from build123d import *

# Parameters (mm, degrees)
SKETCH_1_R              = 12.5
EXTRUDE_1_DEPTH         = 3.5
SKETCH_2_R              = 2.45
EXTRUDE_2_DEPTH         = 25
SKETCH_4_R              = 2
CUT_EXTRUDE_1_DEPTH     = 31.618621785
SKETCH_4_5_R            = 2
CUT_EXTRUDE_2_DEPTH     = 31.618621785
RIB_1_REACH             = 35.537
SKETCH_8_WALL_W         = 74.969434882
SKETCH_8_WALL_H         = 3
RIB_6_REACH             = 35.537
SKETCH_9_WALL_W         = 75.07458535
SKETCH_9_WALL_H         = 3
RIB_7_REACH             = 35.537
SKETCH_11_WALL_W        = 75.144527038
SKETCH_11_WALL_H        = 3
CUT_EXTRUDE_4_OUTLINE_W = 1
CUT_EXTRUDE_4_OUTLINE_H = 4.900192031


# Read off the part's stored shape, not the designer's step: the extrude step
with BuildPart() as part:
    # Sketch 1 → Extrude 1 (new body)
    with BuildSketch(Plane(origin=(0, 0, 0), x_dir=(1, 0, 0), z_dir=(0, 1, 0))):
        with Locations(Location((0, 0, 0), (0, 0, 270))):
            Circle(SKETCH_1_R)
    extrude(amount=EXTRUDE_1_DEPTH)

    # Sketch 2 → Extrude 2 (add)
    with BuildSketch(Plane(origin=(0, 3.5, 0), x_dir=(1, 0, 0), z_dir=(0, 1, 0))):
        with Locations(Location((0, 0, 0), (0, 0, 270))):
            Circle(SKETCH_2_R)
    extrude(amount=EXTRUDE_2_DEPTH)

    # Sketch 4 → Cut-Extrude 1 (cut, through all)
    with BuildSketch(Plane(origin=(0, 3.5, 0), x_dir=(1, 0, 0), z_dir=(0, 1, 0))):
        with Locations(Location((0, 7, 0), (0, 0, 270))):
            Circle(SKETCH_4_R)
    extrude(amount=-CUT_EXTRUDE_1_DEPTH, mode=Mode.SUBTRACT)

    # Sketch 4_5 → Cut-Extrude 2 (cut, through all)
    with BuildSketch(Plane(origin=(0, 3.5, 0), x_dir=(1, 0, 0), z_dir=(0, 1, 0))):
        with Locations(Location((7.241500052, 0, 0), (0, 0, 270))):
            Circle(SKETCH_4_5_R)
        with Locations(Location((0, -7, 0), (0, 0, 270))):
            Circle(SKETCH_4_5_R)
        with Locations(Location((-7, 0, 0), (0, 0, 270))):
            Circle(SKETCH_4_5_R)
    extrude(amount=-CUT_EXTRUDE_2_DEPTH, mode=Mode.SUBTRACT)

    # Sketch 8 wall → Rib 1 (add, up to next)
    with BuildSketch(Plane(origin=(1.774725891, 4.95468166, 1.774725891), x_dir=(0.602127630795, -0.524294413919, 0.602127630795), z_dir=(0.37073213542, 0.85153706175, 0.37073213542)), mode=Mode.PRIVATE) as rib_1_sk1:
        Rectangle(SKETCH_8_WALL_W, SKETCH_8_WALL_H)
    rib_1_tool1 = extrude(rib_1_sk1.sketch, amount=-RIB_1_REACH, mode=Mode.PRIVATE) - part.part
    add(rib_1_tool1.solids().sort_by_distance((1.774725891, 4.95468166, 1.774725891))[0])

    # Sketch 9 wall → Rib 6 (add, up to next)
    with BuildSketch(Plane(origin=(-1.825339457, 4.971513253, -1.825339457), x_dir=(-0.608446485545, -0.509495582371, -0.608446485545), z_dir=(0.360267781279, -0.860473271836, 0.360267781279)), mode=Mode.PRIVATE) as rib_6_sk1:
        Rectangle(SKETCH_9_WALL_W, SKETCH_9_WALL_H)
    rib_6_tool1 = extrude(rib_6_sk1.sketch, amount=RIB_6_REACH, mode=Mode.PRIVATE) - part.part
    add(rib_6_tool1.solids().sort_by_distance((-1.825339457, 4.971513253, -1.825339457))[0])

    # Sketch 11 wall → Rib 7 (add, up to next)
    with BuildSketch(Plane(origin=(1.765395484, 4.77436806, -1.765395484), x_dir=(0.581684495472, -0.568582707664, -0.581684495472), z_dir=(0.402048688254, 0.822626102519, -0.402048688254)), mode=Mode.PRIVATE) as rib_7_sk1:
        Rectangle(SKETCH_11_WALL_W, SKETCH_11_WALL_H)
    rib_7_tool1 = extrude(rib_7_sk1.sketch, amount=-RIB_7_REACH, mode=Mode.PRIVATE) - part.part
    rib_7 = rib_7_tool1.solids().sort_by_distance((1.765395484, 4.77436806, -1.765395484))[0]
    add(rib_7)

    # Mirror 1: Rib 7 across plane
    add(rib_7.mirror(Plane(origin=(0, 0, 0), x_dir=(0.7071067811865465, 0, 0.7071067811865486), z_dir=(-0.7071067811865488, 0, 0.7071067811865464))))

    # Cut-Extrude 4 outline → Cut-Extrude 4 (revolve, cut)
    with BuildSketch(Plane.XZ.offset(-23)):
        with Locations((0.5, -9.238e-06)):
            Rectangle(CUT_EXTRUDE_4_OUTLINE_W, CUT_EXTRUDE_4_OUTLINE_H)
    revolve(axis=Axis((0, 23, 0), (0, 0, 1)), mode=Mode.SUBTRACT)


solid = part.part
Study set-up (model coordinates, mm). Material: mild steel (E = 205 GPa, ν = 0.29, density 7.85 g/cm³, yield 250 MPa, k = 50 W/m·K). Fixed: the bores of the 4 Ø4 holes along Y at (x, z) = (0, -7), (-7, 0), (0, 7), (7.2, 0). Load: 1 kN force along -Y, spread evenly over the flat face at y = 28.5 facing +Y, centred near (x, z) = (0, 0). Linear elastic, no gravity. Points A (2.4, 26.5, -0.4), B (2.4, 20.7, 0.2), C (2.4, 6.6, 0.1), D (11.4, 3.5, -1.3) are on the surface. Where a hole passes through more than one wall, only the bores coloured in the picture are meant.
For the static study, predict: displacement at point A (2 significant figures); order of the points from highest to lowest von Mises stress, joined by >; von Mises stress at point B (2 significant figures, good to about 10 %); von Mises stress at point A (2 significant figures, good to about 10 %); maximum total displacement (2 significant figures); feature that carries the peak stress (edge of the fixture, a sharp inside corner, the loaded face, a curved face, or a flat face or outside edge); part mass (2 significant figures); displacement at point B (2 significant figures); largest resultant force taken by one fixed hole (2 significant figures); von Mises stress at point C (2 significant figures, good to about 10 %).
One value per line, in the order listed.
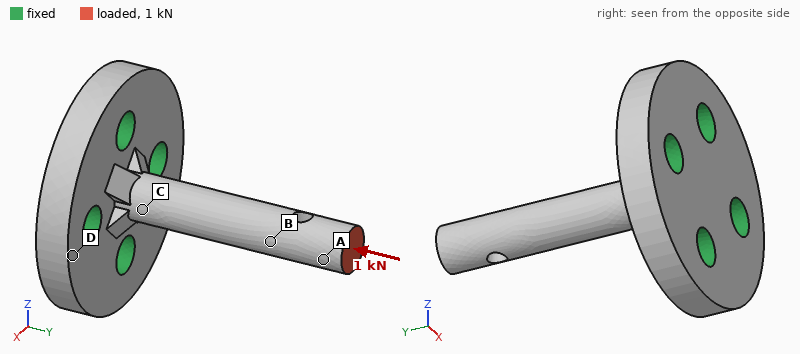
7.5 µm
B > A > C > D
85 MPa
66 MPa
8.1 µm
a curved face
16 g
5.4 µm
270 N
51 MPa
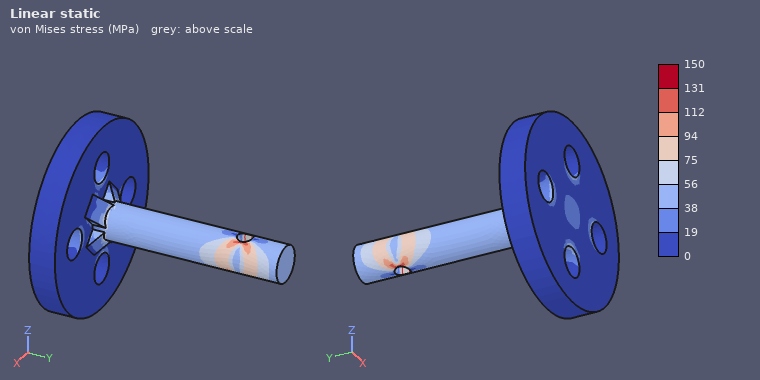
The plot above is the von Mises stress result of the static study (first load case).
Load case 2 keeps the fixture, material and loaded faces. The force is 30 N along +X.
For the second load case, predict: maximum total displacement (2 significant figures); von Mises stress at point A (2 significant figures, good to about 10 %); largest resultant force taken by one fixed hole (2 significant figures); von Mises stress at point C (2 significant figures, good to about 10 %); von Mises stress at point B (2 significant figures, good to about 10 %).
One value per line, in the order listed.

28 µm
5.0 MPa
69 N
55 MPa
23 MPa
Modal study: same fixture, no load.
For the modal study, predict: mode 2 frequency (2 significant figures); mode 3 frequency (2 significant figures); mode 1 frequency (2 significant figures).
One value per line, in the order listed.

5700 Hz
30 kHz
5600 Hz
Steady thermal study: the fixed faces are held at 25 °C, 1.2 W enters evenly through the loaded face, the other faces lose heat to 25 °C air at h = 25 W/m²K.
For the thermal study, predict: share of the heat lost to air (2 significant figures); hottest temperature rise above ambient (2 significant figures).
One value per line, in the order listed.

14 %
32 K
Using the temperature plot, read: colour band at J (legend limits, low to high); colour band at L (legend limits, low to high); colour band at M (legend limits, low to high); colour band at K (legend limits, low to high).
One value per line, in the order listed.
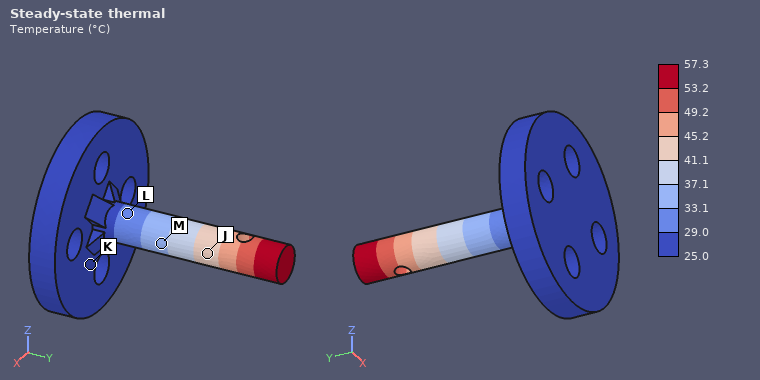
41.1 to 45.2 °C
29.0 to 33.1 °C
33.1 to 37.1 °C
25.0 to 29.0 °C
